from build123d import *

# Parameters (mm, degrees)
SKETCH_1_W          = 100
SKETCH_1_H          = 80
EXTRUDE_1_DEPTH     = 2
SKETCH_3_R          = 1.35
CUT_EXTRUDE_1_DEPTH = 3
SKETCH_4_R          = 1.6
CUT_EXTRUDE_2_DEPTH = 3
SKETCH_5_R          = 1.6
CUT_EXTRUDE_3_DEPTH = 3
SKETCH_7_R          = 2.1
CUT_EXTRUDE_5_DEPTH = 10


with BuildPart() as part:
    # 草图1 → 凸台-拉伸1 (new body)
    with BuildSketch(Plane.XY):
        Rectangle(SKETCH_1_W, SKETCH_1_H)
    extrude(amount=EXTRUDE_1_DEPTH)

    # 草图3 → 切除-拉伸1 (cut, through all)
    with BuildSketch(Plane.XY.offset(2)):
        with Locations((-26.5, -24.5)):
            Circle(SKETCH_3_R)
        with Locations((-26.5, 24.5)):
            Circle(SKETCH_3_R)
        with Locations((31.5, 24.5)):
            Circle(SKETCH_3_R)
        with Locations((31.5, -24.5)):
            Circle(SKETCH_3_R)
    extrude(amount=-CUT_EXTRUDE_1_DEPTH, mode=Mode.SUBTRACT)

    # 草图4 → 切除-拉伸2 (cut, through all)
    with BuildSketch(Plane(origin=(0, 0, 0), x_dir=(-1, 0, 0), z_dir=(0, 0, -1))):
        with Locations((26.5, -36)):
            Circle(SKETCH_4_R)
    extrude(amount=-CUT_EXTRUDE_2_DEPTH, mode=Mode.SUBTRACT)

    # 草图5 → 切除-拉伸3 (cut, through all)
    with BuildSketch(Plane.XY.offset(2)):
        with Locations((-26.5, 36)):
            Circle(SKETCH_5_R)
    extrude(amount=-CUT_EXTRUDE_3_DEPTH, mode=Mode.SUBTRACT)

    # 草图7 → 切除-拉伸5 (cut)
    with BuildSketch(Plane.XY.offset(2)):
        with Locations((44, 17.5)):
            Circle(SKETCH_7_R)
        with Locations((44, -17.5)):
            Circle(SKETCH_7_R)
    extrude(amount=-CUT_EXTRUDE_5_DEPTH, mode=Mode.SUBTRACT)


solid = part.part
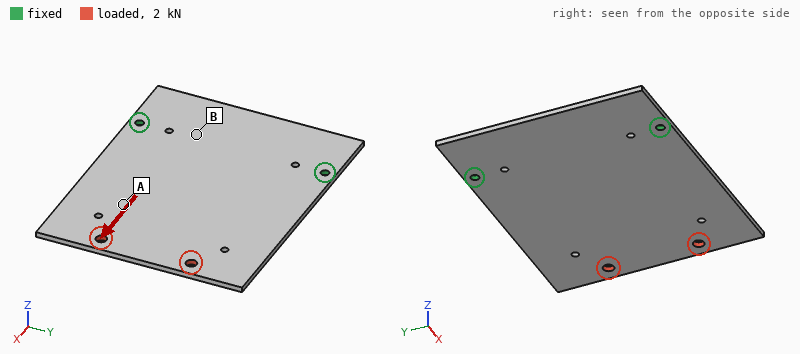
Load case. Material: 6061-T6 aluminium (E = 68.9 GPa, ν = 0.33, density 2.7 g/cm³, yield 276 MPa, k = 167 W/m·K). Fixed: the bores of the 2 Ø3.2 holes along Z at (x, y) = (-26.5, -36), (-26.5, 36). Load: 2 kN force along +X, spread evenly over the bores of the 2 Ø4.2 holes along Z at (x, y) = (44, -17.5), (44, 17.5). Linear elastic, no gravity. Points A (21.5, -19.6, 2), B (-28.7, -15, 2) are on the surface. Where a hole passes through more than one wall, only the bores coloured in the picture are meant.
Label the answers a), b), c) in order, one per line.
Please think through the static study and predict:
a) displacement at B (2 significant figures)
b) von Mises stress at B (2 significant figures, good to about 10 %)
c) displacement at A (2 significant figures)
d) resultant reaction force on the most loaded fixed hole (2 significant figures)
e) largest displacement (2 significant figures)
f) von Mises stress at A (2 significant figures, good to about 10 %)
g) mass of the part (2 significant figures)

a) 9.6 µm
b) 6.0 MPa
c) 16 µm
d) 1.0 kN
e) 26 µm
f) 16 MPa
g) 43 g
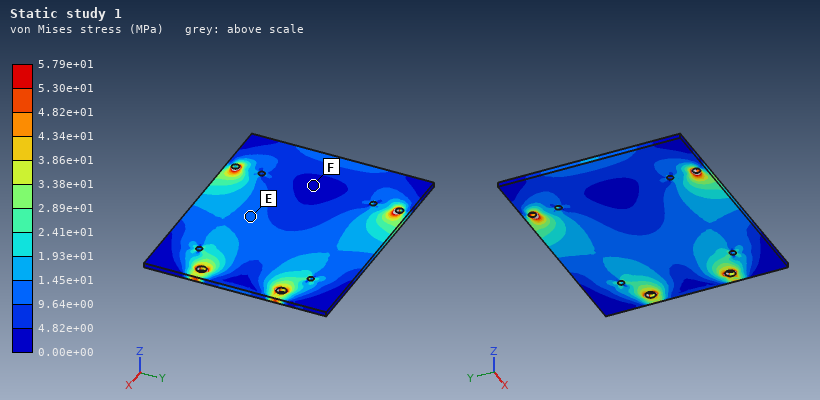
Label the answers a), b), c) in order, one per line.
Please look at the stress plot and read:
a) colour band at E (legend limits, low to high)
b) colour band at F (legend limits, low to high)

a) 9.64e+00 to 1.45e+01 MPa
b) 0.00e+00 to 4.82e+00 MPa
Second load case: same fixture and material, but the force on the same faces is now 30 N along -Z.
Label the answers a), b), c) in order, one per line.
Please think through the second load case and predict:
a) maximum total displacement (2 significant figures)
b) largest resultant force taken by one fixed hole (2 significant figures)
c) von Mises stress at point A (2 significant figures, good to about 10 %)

a) 1.5 mm
b) 15 N
c) 15 MPa
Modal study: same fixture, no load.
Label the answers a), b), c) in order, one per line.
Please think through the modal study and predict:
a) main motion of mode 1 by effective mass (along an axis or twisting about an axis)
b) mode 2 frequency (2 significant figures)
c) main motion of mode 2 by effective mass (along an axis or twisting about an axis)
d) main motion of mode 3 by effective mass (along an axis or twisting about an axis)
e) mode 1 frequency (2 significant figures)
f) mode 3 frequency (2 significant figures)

a) along Z
b) 670 Hz
c) twisting about X
d) along Z
e) 230 Hz
f) 1500 Hz
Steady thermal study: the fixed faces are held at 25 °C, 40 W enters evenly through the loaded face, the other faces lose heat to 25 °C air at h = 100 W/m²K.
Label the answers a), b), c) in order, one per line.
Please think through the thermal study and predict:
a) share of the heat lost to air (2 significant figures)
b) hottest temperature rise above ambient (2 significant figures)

a) 82 %
b) 68 K
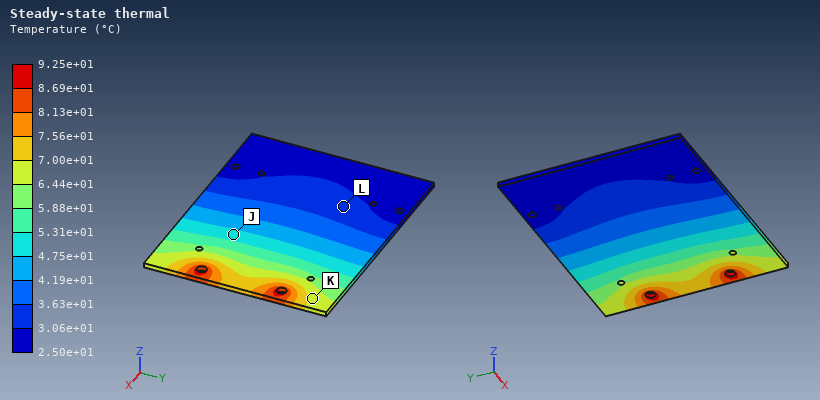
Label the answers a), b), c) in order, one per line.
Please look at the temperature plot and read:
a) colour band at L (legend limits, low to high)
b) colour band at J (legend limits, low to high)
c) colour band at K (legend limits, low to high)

a) 3.06e+01 to 3.63e+01 °C
b) 4.75e+01 to 5.31e+01 °C
c) 6.44e+01 to 7.00e+01 °C
